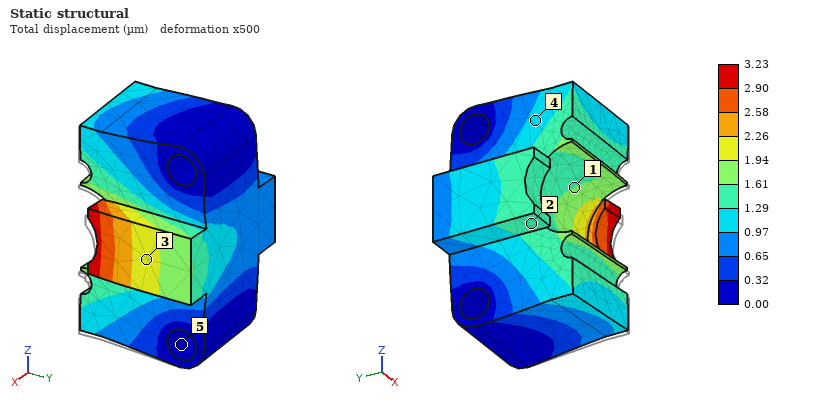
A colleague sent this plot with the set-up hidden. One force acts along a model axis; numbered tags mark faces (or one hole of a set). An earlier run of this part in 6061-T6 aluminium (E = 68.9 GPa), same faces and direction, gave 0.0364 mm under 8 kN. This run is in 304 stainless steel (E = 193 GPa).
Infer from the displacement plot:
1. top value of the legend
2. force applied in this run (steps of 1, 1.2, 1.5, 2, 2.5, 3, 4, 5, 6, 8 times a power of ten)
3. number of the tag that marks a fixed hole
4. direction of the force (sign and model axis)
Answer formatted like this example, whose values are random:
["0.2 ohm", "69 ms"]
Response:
["3.23 µm", "2 kN", "5", "-X"]
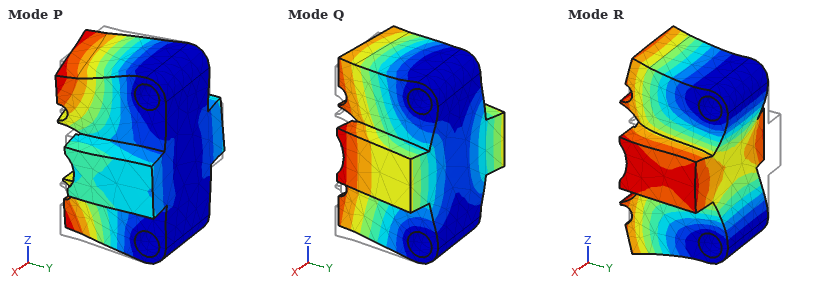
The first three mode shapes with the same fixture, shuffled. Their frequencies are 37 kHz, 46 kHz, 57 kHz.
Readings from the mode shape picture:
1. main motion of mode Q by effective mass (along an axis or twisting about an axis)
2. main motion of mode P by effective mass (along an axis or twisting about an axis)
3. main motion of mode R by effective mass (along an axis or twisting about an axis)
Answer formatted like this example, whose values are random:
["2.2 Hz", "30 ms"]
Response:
["along X", "twisting about Y", "along Y"]
